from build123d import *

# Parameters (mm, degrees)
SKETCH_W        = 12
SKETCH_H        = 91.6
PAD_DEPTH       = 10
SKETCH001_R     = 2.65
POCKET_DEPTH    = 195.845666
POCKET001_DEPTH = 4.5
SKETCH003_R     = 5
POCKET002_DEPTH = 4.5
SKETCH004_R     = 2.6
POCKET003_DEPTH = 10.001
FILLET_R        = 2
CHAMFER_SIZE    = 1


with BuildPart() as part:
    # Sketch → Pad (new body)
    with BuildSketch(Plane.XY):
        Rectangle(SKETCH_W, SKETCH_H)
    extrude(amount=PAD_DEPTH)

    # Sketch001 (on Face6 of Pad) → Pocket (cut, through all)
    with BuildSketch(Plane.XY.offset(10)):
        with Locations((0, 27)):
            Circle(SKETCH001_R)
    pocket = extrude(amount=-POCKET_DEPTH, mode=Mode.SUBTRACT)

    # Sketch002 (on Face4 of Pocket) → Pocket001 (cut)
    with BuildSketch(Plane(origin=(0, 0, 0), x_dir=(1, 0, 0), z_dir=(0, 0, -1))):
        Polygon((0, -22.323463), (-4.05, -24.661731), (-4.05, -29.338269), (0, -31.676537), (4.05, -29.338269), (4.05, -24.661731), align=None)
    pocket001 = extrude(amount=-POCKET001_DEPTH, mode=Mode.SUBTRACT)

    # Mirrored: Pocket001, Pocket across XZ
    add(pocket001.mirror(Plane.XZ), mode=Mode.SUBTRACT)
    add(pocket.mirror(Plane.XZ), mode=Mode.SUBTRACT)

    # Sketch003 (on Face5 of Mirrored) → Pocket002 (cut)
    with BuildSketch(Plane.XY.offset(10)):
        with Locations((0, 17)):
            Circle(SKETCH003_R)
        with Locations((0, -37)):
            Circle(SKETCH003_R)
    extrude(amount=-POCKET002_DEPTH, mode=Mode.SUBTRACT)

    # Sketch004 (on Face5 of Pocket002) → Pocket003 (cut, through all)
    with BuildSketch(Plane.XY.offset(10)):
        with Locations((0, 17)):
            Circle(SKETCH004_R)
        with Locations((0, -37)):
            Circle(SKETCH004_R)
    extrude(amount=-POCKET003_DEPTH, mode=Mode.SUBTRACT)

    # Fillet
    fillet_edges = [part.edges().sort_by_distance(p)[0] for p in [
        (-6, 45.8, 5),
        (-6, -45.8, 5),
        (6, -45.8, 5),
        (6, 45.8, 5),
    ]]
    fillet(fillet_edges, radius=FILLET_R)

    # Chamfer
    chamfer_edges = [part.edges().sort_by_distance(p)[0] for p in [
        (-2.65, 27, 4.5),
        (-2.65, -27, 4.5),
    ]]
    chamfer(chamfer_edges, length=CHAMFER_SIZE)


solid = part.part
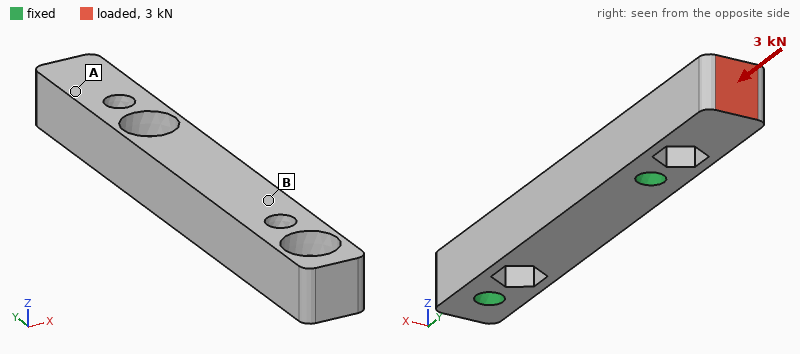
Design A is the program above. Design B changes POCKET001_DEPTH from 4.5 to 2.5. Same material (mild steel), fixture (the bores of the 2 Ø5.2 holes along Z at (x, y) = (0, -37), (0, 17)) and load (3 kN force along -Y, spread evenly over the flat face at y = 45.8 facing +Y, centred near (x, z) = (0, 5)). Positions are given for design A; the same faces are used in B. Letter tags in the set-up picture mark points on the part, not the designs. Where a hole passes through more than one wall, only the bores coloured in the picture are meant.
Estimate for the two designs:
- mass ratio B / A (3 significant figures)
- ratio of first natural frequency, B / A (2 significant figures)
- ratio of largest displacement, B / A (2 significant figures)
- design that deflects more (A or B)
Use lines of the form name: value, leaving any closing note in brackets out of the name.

mass ratio B / A: 1.02
ratio of first natural frequency, B / A: 1.0
ratio of largest displacement, B / A: 1.1
design that deflects more: B
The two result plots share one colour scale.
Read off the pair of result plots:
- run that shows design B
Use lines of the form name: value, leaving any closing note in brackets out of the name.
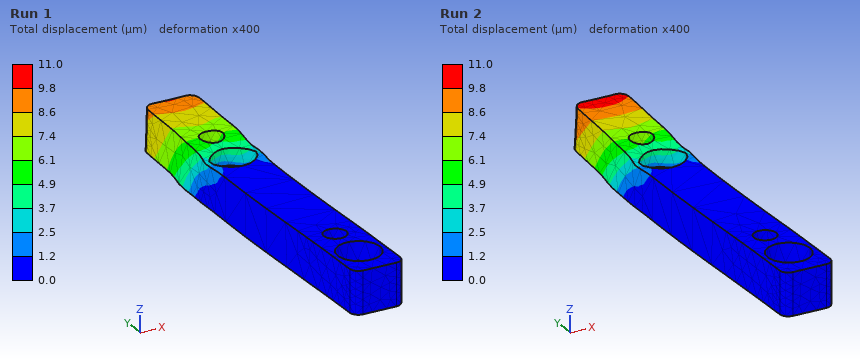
run that shows design B: Run 2
